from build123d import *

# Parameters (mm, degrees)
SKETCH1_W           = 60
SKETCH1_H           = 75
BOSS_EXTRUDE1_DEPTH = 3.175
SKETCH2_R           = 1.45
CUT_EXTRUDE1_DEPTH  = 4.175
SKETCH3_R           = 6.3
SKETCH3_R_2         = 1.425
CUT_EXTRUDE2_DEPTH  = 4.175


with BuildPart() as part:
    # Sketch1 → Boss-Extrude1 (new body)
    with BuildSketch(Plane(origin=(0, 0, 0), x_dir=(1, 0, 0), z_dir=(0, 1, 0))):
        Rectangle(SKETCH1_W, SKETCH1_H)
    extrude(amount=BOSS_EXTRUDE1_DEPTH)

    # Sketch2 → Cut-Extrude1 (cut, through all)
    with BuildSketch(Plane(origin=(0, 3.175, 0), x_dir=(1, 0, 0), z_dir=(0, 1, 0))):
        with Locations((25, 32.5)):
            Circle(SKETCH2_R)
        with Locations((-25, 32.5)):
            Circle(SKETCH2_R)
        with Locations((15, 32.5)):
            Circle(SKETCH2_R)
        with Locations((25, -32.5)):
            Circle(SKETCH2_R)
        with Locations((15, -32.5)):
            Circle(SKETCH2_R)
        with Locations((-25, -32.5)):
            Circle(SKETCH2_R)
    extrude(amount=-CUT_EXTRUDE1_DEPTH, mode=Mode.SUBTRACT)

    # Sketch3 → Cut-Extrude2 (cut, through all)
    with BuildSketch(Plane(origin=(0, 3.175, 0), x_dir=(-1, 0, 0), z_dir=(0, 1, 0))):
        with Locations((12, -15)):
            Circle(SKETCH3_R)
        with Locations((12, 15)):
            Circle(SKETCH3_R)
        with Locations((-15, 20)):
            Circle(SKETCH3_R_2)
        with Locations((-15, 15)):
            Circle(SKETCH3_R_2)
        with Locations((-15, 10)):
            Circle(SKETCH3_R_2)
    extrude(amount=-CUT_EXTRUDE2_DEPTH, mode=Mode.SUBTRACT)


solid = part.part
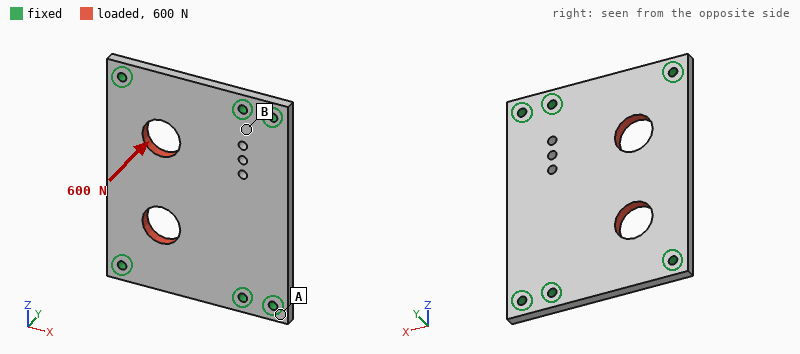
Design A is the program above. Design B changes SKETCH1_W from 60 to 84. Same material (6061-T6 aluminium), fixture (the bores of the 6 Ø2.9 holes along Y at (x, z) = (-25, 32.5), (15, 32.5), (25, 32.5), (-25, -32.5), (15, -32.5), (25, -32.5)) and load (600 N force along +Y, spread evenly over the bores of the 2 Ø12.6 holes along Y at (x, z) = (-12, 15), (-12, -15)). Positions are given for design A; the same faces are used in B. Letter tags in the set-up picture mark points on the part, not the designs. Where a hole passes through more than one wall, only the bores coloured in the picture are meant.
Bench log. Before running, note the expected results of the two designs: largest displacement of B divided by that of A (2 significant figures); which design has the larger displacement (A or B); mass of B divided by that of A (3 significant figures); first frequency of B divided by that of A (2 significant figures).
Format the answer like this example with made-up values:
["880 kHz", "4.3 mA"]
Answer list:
["0.88", "A", "1.43", "0.95"]
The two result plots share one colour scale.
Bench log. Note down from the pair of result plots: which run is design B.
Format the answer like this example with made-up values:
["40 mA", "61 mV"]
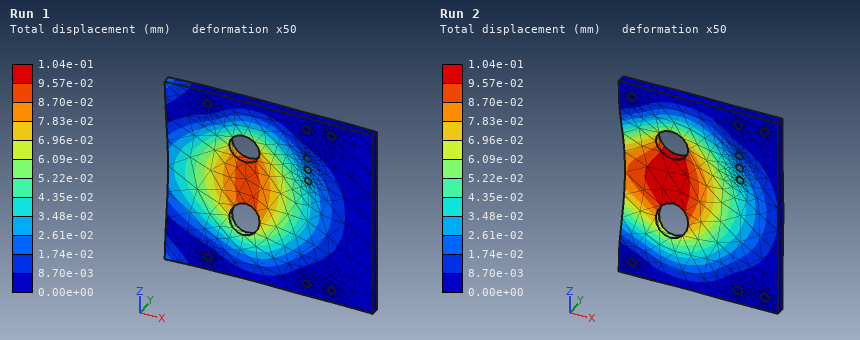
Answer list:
["Run 1"]
